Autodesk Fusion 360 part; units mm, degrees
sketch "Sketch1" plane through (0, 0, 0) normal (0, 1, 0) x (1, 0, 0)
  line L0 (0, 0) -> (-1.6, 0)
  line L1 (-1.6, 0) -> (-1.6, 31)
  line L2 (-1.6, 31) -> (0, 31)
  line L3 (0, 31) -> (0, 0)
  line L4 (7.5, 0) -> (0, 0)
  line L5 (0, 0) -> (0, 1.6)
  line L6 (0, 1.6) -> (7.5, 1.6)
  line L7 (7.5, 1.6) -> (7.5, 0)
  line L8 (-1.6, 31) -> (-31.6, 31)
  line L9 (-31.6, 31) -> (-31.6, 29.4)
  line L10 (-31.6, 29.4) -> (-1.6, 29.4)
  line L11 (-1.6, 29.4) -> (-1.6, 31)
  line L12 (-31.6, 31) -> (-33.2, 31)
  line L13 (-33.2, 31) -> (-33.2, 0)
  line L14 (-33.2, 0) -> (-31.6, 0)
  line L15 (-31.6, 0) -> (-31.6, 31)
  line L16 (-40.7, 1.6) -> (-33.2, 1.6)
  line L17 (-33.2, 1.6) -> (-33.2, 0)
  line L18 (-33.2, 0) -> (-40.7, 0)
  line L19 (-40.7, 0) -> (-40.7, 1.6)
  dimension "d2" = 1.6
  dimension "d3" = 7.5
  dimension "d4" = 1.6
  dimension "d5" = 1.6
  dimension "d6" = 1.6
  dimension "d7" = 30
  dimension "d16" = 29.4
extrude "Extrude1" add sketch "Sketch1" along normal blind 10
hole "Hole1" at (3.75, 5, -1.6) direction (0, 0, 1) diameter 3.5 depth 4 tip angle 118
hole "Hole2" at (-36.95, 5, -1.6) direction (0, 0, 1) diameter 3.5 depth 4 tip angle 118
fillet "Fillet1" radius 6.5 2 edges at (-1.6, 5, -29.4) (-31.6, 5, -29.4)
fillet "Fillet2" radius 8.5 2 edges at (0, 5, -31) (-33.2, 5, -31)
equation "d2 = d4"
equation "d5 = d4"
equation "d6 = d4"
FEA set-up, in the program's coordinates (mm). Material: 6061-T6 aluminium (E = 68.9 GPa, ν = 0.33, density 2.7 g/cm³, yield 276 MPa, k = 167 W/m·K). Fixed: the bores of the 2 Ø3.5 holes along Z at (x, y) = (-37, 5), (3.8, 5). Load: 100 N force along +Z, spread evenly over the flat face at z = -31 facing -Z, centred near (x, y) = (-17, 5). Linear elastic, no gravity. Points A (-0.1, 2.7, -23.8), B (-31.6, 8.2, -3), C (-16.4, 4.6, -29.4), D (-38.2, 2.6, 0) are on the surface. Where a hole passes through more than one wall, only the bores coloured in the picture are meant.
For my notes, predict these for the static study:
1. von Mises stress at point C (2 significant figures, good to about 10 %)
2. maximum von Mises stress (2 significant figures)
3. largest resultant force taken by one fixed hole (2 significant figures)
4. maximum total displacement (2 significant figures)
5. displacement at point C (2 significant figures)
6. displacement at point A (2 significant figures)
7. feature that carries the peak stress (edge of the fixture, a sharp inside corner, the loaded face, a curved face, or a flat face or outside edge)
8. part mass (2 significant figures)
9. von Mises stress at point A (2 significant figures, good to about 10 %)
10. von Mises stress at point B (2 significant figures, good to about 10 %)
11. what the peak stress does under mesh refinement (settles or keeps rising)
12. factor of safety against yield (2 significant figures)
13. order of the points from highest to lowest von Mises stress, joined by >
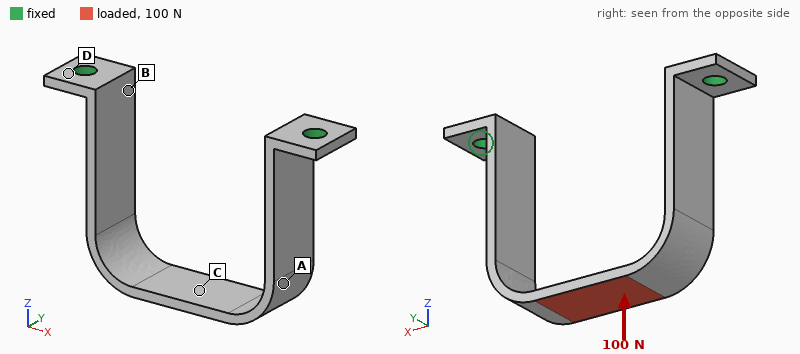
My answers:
67 MPa
72 MPa
52 N
98 µm
93 µm
36 µm
the loaded face
4.2 g
38 MPa
20 MPa
settles
3.8
C > A > B > D
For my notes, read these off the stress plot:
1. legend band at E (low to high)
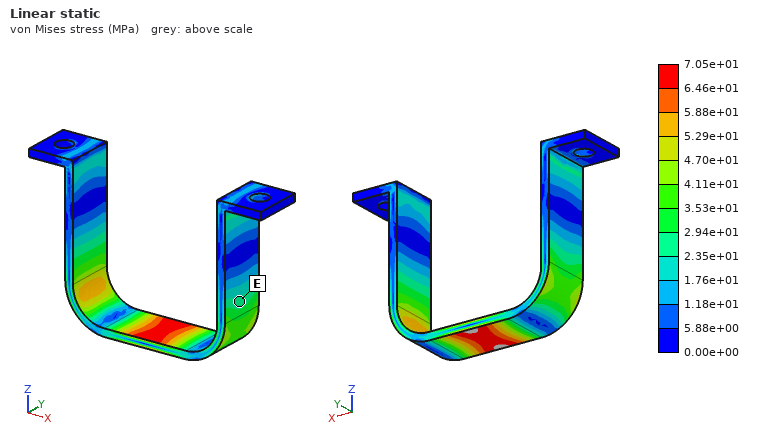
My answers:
2.35e+01 to 2.94e+01 MPa
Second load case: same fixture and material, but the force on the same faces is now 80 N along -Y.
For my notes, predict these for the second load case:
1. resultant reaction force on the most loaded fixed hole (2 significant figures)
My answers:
40 N
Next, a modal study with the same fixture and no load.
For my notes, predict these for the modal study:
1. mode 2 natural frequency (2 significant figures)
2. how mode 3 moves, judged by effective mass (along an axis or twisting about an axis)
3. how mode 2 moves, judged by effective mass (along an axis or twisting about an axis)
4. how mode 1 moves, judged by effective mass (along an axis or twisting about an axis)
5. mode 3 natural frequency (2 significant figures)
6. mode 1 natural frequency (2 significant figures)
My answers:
2100 Hz
twisting about Z
along Y
along X
3400 Hz
1400 Hz
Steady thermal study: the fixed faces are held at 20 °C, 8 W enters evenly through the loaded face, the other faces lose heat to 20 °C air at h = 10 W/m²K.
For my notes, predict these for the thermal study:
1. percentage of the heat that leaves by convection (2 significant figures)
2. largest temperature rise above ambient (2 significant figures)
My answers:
7.2 %
60 K
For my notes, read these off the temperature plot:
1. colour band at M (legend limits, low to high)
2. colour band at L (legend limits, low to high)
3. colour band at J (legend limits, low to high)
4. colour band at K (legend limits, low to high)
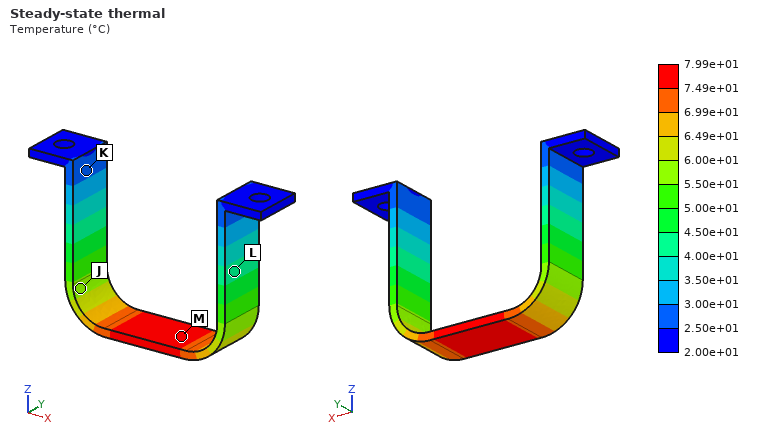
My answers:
7.49e+01 to 7.99e+01 °C
4.00e+01 to 4.50e+01 °C
5.50e+01 to 6.00e+01 °C
2.50e+01 to 3.00e+01 °C
